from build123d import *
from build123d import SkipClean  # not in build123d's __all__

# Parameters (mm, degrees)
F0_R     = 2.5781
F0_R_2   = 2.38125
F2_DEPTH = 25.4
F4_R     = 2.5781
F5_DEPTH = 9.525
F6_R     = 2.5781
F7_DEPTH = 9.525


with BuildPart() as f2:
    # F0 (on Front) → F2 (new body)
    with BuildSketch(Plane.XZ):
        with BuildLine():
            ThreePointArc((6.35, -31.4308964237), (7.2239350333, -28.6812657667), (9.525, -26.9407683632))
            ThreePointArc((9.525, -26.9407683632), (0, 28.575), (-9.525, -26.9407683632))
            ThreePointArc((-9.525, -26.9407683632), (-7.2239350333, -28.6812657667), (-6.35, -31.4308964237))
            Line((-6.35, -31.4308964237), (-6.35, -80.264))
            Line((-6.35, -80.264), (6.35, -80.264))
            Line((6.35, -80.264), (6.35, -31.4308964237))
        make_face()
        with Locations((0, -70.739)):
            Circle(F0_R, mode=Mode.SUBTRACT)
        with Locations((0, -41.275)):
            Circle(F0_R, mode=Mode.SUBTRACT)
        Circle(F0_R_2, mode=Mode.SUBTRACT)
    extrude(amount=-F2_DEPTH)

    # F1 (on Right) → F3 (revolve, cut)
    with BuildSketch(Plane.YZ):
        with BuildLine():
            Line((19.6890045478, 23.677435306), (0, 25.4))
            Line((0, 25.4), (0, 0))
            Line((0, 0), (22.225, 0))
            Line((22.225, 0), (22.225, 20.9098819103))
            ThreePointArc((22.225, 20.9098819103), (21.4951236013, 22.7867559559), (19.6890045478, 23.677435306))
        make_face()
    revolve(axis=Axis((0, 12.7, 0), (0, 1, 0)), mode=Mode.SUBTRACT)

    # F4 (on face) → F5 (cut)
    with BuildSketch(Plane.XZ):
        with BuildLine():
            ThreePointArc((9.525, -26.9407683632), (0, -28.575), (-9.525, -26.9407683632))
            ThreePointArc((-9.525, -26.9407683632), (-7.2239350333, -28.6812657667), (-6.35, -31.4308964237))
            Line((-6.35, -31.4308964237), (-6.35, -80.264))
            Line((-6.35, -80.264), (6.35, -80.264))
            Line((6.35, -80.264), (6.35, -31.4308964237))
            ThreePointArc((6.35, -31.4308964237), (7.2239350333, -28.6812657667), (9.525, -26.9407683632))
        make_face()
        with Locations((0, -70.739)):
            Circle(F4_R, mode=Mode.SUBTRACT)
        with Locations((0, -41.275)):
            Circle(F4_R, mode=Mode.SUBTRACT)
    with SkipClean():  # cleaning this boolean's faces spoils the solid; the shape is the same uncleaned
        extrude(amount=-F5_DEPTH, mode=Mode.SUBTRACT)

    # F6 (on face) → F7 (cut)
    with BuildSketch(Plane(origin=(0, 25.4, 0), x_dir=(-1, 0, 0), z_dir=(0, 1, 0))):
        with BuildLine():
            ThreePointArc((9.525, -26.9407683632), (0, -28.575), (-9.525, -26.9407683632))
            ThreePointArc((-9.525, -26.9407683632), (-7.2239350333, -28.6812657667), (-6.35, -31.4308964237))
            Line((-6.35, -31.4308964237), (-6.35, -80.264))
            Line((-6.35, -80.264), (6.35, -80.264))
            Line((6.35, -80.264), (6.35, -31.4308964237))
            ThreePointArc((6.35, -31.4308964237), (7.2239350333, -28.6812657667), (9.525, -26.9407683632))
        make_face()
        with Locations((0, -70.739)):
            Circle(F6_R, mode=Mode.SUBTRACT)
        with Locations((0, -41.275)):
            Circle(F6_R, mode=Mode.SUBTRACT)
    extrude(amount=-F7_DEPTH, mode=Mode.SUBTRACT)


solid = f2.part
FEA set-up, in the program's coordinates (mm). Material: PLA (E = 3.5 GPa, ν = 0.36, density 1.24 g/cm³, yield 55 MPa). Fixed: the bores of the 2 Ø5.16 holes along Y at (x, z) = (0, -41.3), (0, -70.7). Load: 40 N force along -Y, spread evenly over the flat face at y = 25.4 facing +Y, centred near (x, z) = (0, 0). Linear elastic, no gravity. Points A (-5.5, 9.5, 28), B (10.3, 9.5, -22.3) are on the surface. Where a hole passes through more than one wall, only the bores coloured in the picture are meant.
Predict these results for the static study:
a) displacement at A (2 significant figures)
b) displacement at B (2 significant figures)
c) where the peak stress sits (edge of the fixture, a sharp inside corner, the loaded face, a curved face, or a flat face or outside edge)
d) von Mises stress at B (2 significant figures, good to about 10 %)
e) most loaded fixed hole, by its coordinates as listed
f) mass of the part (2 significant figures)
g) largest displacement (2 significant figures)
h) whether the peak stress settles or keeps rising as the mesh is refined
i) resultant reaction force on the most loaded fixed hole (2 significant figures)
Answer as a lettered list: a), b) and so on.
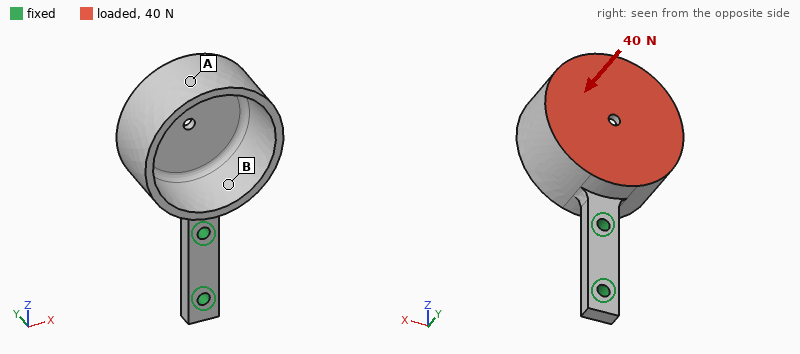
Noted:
a) 1.4 mm
b) 0.23 mm
c) edge of the fixture
d) 3.2 MPa
e) (0, -41.3)
f) 34 g
g) 1.4 mm
h) keeps rising
i) 43 N
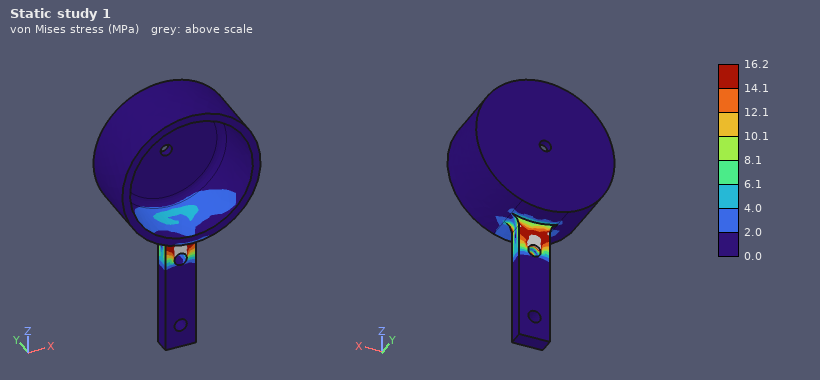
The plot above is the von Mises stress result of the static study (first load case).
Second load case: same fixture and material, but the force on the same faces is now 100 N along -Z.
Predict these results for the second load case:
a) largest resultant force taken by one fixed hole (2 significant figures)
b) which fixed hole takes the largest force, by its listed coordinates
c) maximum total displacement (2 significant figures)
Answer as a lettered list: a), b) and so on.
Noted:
a) 97 N
b) (0, -41.3)
c) 1.3 mm
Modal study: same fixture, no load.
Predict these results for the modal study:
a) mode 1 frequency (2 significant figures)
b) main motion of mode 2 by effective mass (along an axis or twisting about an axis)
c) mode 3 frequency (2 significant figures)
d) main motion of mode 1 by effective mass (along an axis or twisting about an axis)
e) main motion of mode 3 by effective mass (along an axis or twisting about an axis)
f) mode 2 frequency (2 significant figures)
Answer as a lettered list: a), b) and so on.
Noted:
a) 190 Hz
b) along X
c) 420 Hz
d) along Y
e) twisting about Z
f) 260 Hz
